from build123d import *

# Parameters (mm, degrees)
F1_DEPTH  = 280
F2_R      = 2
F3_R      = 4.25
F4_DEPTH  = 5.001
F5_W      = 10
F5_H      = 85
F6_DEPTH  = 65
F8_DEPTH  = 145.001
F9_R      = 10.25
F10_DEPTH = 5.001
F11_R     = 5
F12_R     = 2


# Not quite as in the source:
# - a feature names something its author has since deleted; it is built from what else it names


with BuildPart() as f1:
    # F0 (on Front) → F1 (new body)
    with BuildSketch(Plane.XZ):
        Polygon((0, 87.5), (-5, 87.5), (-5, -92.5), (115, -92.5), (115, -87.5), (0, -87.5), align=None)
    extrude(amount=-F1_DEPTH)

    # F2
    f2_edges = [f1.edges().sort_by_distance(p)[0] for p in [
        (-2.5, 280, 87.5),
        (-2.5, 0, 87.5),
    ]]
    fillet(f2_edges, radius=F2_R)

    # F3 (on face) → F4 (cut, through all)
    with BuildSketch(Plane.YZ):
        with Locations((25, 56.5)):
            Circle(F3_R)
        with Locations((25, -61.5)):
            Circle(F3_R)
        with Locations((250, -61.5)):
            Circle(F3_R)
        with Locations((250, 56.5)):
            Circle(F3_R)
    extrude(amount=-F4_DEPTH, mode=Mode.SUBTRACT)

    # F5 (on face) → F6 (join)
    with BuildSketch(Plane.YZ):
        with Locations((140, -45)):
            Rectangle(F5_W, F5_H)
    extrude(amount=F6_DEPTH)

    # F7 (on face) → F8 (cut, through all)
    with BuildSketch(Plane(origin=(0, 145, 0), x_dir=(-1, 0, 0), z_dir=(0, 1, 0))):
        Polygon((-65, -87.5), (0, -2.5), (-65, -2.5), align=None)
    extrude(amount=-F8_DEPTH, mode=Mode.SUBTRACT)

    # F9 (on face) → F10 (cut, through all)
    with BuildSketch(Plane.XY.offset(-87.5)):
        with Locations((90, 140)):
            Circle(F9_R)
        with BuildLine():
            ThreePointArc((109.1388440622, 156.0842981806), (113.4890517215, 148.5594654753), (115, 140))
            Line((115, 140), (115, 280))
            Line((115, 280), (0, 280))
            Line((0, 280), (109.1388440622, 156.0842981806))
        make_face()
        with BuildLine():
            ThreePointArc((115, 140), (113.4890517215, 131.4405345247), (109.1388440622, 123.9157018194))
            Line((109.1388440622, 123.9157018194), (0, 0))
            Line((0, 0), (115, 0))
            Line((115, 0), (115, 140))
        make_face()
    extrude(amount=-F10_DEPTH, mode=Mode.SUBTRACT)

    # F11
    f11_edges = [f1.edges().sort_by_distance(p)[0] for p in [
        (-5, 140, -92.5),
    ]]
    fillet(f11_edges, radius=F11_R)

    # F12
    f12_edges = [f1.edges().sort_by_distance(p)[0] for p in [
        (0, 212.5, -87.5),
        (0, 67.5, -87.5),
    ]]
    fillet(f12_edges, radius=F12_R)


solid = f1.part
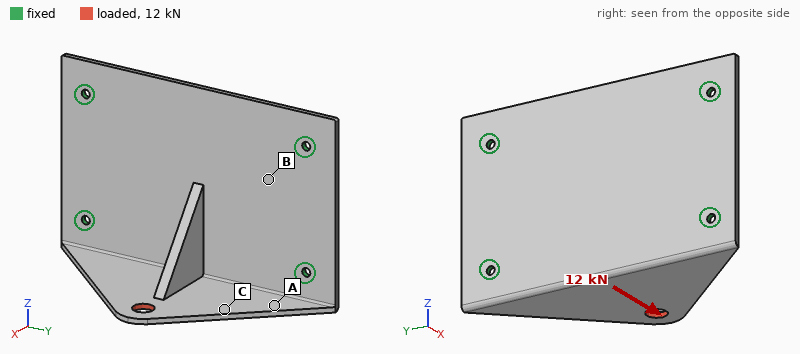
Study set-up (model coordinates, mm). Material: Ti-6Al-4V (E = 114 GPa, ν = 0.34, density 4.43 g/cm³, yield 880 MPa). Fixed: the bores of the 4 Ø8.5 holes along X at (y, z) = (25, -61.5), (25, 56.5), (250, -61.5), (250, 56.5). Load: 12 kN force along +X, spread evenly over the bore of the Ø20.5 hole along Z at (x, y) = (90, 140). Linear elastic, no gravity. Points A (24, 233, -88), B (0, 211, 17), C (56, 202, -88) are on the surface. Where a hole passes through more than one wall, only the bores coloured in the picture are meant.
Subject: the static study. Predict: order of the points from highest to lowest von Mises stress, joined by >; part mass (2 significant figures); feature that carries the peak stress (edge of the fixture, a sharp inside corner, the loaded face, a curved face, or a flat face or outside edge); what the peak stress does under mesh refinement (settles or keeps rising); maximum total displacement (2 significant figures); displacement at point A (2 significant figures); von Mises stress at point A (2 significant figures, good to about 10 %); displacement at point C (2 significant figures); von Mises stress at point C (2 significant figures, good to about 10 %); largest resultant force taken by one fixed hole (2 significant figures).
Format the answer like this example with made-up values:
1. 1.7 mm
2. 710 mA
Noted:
1. A > C > B
2. 1.6 kg
3. edge of the fixture
4. keeps rising
5. 1.2 mm
6. 0.72 mm
7. 110 MPa
8. 0.91 mm
9. 60 MPa
10. 8.3 kN
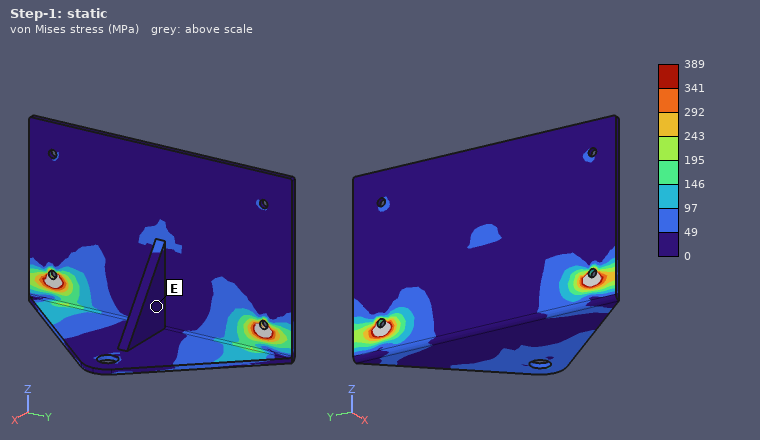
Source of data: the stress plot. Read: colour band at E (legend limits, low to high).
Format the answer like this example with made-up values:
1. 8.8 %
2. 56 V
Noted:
1. 0 to 49 MPa
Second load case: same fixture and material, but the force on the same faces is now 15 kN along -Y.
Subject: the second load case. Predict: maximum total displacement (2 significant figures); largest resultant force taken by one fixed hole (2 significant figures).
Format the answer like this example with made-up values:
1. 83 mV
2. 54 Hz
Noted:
1. 0.78 mm
2. 9.5 kN
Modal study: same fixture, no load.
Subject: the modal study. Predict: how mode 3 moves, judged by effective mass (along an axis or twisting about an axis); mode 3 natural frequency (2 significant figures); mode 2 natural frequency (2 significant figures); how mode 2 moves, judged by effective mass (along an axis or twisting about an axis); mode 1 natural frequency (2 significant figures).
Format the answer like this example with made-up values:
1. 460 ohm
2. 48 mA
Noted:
1. along X
2. 950 Hz
3. 790 Hz
4. along X
5. 450 Hz
